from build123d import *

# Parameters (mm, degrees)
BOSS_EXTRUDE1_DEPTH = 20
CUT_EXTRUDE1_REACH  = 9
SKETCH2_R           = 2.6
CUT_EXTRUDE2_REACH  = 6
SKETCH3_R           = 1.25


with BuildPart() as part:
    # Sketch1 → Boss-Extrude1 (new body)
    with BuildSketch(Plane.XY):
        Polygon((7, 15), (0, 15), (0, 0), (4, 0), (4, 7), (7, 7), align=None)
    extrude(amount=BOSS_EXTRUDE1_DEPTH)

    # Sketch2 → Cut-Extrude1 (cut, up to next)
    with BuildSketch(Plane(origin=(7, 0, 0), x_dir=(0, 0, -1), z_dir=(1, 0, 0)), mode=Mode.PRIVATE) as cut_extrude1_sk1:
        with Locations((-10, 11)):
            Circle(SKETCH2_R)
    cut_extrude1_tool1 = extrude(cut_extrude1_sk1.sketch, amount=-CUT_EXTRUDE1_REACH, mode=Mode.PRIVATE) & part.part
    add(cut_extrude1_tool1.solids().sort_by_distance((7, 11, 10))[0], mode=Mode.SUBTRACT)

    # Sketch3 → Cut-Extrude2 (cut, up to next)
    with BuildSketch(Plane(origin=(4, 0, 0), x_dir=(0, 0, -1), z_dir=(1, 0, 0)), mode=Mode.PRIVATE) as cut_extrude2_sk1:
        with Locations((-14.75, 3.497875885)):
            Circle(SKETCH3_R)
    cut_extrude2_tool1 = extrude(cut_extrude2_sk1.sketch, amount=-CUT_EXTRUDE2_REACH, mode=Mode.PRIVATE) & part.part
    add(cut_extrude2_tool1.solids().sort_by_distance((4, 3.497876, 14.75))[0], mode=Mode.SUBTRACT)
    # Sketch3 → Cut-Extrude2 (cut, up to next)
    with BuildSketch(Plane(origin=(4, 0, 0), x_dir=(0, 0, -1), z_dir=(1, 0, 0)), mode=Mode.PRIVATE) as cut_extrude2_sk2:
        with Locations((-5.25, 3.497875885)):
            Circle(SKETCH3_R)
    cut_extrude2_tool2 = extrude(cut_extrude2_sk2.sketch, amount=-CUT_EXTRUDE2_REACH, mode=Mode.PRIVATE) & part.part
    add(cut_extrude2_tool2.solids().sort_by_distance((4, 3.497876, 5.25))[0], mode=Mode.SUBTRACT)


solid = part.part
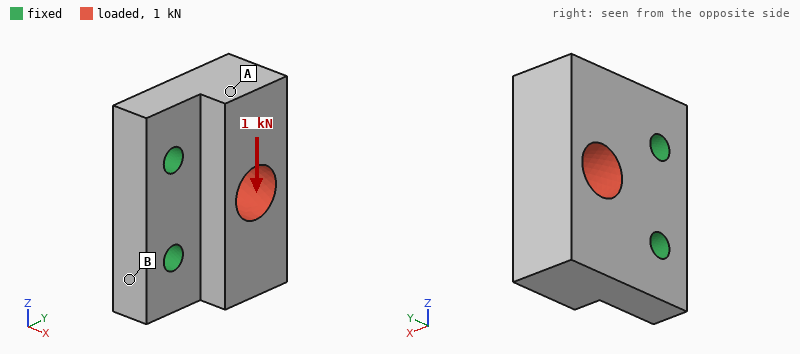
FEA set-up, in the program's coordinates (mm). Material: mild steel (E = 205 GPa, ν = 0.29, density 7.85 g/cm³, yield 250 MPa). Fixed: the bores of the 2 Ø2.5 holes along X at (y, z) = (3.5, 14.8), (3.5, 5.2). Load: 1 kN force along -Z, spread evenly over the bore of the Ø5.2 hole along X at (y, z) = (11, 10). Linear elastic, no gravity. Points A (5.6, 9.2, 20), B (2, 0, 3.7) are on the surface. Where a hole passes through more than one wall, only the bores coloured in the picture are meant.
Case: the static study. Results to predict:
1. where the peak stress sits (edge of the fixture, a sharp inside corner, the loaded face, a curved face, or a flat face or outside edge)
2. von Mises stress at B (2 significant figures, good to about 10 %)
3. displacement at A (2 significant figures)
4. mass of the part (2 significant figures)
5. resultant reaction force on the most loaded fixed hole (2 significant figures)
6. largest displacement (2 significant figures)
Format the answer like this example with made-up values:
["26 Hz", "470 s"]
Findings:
["edge of the fixture", "21 MPa", "2.5 µm", "12 g", "780 N", "4.0 µm"]
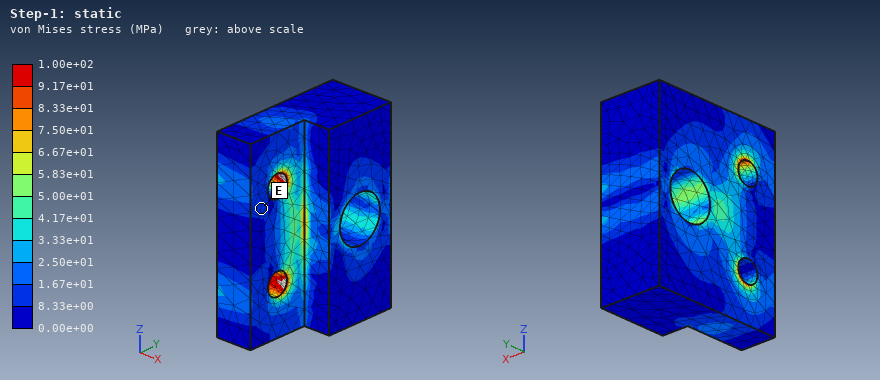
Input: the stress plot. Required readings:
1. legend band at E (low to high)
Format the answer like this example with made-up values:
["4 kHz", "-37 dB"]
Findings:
["8.33e+00 to 1.67e+01 MPa"]
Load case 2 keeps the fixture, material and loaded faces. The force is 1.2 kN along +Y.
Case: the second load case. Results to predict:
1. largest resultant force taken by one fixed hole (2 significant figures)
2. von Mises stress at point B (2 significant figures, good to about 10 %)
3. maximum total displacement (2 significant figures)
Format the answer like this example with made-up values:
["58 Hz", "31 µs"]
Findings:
["620 N", "10 MPa", "5.7 µm"]
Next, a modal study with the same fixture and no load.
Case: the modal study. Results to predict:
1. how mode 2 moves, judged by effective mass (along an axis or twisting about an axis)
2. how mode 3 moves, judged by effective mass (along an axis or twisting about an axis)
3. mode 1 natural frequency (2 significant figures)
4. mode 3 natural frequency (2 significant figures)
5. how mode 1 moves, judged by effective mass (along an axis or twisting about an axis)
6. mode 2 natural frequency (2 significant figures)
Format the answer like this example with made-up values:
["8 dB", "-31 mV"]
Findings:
["twisting about Y", "along Z", "18 kHz", "33 kHz", "along X", "28 kHz"]
